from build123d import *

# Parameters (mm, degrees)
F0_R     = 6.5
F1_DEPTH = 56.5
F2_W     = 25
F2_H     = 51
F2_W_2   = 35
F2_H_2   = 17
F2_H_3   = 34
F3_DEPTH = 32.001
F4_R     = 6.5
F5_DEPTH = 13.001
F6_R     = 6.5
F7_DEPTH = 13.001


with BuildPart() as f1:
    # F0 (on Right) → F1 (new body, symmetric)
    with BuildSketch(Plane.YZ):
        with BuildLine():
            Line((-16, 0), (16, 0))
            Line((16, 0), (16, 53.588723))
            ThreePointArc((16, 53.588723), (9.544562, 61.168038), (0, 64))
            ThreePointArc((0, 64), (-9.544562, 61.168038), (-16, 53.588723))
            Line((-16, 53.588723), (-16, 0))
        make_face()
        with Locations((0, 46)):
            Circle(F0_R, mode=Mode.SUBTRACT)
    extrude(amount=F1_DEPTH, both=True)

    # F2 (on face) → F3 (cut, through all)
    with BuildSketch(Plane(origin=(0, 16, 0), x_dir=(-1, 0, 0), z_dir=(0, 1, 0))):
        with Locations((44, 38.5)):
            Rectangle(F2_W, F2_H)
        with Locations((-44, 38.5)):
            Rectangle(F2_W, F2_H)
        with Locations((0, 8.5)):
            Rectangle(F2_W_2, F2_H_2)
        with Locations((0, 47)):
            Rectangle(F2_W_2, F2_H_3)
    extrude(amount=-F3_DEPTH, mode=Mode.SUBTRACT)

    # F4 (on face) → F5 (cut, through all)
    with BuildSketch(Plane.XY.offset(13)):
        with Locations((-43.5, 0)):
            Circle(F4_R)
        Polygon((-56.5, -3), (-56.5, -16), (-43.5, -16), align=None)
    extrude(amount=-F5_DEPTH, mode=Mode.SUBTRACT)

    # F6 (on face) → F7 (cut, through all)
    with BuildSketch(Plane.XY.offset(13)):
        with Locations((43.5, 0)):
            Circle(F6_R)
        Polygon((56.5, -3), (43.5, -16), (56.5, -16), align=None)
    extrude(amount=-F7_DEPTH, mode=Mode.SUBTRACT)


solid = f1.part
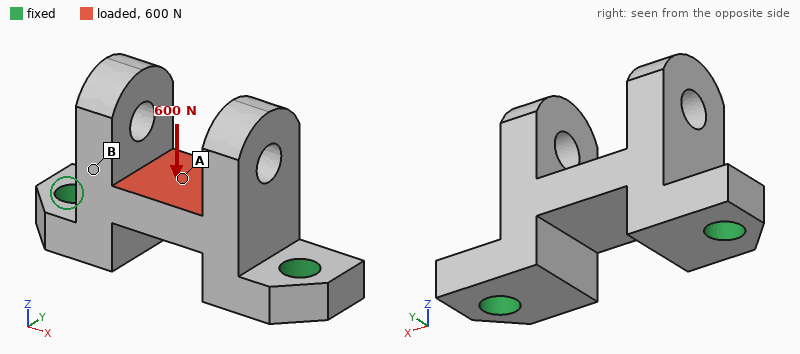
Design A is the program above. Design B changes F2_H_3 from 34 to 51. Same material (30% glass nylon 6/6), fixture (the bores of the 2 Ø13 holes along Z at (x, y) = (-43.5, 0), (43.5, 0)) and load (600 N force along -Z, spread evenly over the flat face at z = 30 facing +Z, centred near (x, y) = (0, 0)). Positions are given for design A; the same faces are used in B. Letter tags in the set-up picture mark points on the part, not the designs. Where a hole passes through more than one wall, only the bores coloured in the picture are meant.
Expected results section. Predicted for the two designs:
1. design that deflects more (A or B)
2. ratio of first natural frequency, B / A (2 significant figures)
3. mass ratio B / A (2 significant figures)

B
0.88
0.88
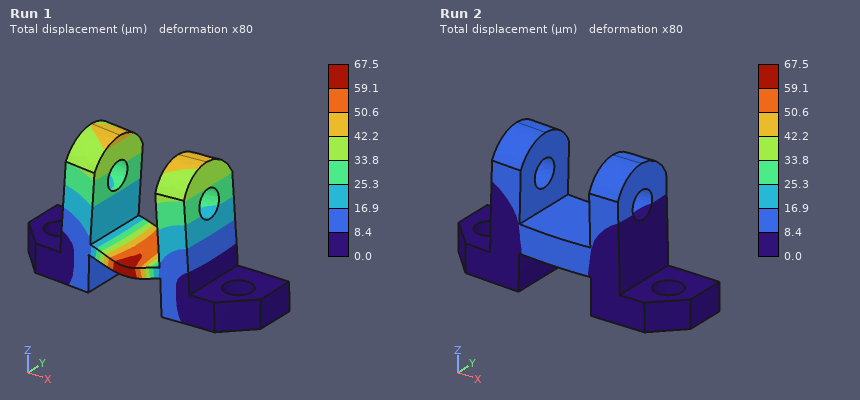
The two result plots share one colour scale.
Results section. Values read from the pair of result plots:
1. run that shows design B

Run 1
